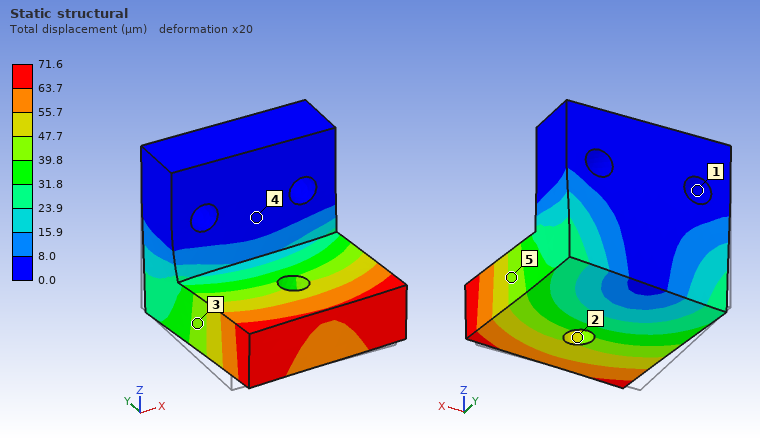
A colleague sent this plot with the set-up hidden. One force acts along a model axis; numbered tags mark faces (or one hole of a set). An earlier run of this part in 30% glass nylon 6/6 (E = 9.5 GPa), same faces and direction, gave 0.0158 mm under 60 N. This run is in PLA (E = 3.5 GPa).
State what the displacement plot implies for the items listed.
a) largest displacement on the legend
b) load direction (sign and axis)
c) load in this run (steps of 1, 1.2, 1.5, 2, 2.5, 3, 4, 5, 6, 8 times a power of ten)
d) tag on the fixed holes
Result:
71.6 µm
+X
100 N
1
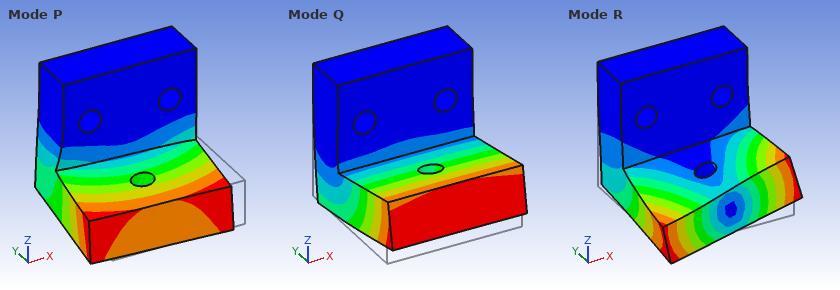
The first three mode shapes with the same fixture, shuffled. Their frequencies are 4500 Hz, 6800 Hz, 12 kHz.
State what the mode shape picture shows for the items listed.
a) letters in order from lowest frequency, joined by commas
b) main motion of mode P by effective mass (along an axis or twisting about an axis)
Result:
Q, P, R
along X
